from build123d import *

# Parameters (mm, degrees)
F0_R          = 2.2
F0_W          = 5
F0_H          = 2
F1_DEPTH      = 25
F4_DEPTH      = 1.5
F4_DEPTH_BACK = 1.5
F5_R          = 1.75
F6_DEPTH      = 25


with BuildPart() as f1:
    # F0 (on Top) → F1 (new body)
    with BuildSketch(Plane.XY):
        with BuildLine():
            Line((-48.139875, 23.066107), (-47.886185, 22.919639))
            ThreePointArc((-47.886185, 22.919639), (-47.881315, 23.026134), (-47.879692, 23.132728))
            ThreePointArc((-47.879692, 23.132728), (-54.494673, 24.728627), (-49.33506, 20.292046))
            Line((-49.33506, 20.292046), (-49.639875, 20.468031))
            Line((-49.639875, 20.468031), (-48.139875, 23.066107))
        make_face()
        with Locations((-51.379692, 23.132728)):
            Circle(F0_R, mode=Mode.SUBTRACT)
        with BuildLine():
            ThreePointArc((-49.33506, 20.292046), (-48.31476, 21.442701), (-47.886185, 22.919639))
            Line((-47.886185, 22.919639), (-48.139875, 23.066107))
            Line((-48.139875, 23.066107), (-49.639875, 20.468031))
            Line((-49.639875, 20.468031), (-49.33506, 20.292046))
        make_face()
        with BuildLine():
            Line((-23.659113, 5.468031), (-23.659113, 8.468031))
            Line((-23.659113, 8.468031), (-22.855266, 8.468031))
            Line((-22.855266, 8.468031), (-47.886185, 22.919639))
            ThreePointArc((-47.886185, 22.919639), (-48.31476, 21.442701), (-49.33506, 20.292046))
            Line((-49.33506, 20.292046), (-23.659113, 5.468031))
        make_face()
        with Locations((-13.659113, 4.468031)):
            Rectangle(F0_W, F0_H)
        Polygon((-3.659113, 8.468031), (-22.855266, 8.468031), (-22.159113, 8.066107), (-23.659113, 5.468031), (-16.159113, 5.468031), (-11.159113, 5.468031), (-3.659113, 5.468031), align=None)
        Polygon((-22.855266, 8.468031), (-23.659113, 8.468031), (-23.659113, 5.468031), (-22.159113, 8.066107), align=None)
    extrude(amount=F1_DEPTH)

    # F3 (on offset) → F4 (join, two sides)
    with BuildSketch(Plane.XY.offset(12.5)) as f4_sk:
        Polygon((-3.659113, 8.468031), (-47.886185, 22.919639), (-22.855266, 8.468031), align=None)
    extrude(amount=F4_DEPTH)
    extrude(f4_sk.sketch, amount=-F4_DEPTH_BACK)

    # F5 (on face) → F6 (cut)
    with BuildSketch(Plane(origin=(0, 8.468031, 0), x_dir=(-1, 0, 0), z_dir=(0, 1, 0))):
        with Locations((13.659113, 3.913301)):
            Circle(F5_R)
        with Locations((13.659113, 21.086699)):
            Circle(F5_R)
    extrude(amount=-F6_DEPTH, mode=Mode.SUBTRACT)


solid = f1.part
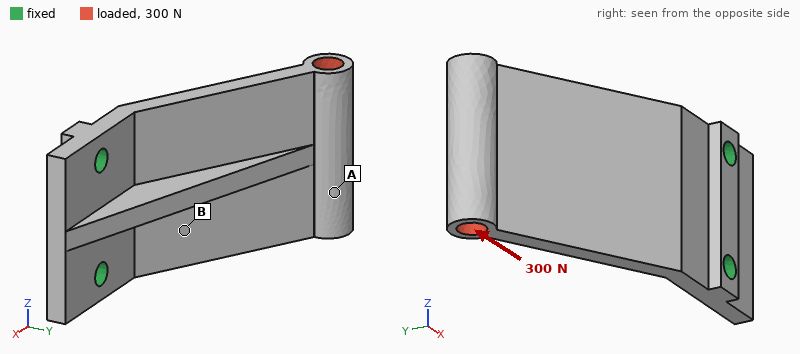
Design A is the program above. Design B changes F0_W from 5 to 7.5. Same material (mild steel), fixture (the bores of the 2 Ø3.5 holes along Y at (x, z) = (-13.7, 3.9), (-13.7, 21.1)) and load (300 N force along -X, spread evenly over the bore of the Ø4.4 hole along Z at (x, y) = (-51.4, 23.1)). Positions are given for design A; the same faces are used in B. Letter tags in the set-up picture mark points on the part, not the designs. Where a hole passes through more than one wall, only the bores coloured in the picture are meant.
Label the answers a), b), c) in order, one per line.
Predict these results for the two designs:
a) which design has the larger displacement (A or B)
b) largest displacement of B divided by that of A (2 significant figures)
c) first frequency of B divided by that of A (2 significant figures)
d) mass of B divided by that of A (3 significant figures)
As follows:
a) A
b) 0.92
c) 1.1
d) 1.03
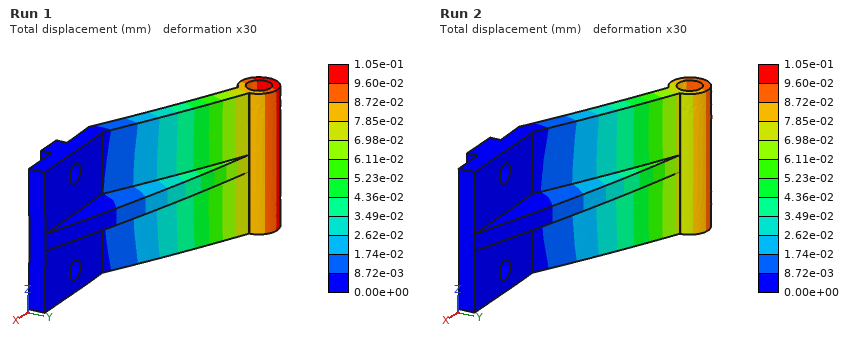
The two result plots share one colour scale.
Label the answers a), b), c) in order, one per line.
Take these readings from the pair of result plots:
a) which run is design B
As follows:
a) Run 2
